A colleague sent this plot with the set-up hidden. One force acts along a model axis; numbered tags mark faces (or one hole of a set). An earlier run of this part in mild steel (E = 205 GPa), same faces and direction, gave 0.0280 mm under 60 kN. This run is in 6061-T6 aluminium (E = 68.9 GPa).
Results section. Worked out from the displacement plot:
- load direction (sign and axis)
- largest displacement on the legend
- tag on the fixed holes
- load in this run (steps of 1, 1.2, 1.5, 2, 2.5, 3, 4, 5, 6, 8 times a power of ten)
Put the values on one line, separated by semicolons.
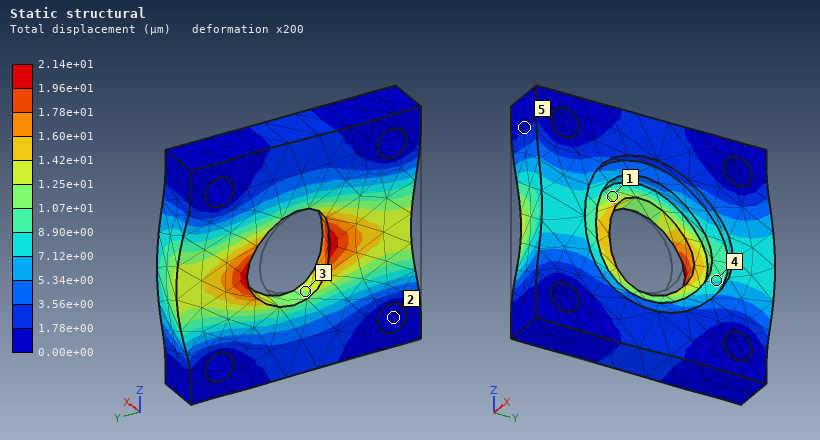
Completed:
+Y; 2.14e+01 µm; 2; 15 kN
